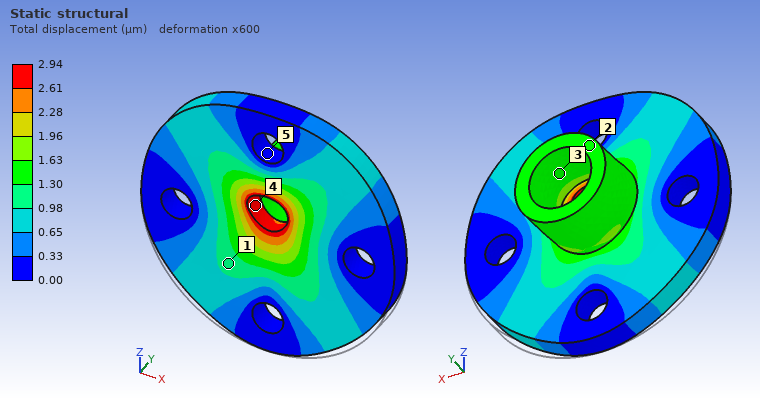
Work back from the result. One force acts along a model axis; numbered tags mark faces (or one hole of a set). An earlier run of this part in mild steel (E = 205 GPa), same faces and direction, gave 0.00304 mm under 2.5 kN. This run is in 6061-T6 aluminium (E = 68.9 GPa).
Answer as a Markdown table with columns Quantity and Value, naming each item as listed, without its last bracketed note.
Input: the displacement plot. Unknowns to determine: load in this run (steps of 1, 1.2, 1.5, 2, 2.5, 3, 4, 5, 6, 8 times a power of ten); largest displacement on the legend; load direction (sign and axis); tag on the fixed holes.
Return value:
| Quantity | Value |
|---|---|
| load in this run | 800 N |
| largest displacement on the legend | 2.94 µm |
| load direction | +Z |
| tag on the fixed holes | 5 |
